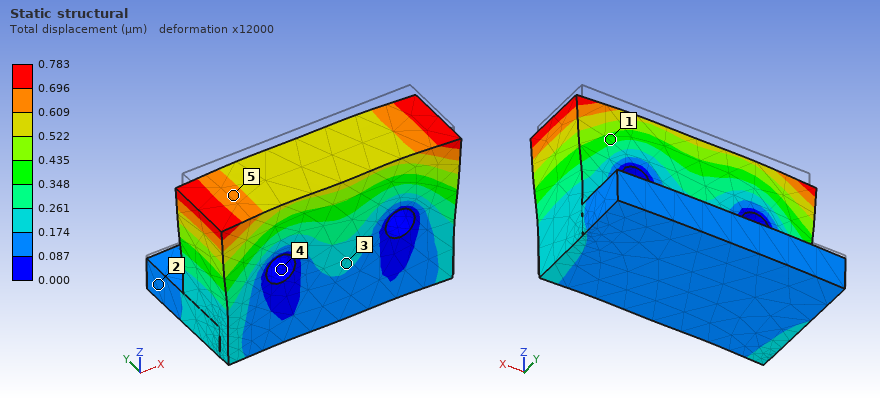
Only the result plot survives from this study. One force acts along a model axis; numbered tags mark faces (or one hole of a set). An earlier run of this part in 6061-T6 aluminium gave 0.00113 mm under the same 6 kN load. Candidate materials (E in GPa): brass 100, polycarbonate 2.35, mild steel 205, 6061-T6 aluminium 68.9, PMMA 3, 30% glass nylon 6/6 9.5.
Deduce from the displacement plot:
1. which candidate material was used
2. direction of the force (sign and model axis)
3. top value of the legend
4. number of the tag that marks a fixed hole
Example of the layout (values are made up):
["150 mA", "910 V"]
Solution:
["brass", "-Z", "0.783 µm", "4"]
